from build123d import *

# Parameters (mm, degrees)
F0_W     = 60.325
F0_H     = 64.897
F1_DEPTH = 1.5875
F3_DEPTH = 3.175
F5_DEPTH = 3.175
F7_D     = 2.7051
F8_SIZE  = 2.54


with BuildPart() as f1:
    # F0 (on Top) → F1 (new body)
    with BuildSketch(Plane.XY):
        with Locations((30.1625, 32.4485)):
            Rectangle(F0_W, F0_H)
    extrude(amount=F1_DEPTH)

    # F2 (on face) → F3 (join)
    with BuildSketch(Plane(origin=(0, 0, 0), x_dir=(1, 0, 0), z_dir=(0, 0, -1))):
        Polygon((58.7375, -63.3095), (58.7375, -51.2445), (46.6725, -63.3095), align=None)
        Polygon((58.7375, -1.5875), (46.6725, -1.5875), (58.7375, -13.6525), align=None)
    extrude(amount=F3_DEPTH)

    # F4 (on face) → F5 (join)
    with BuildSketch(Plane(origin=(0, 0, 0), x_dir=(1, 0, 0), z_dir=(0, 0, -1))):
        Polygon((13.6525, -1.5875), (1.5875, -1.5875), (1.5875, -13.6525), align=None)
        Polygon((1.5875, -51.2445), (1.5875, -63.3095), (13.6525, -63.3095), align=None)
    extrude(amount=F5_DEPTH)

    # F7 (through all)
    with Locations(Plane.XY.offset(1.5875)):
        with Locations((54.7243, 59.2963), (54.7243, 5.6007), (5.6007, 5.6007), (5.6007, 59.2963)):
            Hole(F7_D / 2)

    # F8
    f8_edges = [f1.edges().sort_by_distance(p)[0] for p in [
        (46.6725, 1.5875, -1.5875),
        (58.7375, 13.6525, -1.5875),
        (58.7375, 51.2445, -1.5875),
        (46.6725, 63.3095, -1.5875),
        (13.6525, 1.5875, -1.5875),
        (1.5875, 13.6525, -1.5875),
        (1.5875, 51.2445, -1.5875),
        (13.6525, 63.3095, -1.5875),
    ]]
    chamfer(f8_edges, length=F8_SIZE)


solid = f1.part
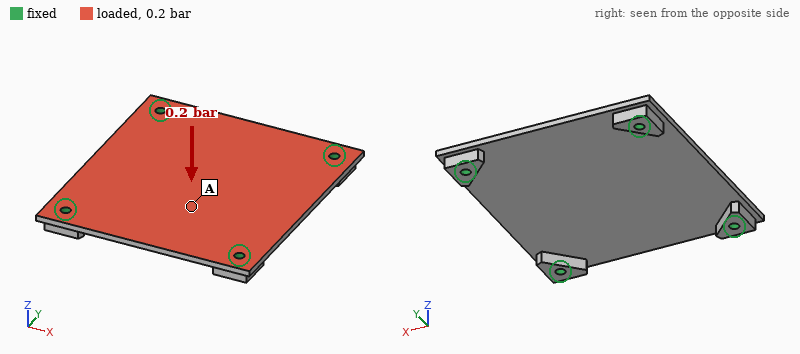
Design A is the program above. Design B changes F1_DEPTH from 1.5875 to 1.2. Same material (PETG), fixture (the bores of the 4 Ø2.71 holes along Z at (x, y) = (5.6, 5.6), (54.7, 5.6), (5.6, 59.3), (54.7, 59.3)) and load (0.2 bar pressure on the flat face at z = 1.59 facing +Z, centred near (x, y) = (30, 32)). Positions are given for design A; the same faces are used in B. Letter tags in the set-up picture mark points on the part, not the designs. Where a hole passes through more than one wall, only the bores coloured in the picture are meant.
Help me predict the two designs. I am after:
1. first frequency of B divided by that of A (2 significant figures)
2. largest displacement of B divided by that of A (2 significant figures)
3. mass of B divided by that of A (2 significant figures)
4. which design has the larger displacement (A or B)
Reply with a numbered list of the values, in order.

1. 0.78
2. 2.2
3. 0.78
4. B
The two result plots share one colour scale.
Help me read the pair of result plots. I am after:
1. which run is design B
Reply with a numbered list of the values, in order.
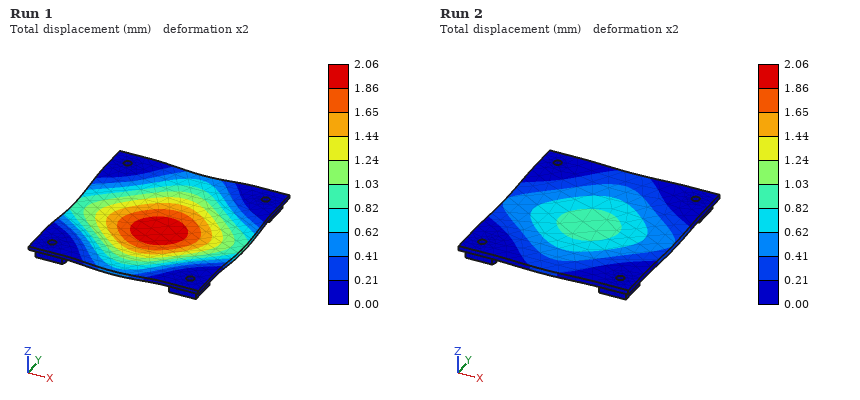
1. Run 1
